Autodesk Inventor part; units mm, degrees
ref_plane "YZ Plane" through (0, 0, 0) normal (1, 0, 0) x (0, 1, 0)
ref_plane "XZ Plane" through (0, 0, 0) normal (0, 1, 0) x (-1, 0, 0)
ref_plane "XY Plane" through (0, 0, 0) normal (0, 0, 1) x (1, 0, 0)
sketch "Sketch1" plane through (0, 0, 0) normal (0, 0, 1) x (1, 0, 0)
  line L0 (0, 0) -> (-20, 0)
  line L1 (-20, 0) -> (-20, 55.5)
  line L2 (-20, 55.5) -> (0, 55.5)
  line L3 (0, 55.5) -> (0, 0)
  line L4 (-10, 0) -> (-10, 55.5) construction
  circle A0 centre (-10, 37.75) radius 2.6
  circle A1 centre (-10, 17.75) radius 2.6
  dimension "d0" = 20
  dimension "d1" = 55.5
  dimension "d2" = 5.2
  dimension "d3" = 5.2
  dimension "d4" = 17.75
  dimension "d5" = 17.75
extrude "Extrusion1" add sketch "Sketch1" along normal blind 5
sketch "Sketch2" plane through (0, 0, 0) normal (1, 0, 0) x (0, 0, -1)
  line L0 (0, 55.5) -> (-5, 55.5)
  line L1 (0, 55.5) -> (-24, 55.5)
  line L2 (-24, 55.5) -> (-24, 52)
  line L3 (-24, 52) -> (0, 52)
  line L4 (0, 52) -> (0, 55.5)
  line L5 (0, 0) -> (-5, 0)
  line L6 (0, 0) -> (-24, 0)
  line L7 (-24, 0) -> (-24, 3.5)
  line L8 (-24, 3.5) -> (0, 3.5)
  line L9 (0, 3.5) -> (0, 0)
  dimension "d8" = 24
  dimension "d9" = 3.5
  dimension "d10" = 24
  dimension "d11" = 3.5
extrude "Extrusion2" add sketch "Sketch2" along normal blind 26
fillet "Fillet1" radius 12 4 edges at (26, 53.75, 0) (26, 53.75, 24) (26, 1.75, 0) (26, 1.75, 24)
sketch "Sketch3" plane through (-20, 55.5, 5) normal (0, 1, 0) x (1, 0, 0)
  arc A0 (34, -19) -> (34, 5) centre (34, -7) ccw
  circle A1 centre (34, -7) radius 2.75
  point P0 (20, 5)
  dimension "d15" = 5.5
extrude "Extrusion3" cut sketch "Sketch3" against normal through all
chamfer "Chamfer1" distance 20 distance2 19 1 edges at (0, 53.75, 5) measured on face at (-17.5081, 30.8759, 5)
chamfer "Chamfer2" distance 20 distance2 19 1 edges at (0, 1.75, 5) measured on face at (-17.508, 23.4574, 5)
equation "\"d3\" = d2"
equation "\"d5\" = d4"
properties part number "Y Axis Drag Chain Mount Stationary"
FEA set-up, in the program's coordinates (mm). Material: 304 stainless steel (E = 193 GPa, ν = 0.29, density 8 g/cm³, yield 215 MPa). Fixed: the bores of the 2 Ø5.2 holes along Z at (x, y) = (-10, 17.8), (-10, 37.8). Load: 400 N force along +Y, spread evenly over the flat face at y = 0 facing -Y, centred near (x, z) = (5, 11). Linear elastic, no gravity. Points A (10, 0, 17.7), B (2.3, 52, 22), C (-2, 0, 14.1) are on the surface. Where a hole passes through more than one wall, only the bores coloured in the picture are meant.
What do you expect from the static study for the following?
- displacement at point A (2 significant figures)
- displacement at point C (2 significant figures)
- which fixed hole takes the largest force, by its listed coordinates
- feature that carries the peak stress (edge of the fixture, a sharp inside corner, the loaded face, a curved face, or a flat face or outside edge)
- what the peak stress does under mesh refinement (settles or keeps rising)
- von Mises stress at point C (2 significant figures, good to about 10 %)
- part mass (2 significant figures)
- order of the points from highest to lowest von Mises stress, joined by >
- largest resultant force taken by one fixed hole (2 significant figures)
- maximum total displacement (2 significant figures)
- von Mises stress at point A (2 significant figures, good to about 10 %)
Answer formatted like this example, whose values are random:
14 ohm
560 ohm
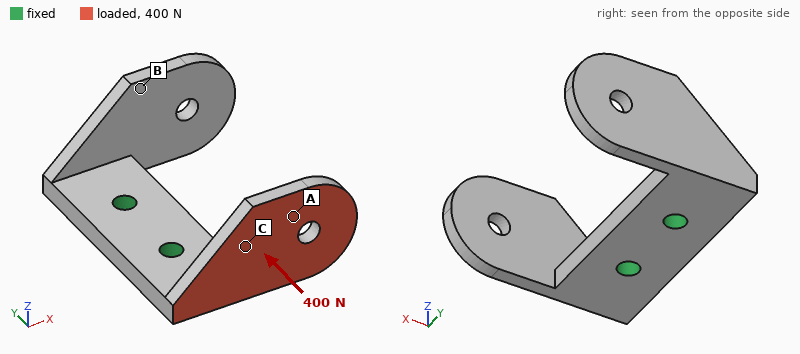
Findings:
0.075 mm
0.034 mm
(-10, 17.8)
a sharp inside corner
keeps rising
53 MPa
83 g
C > A > B
390 N
0.12 mm
19 MPa
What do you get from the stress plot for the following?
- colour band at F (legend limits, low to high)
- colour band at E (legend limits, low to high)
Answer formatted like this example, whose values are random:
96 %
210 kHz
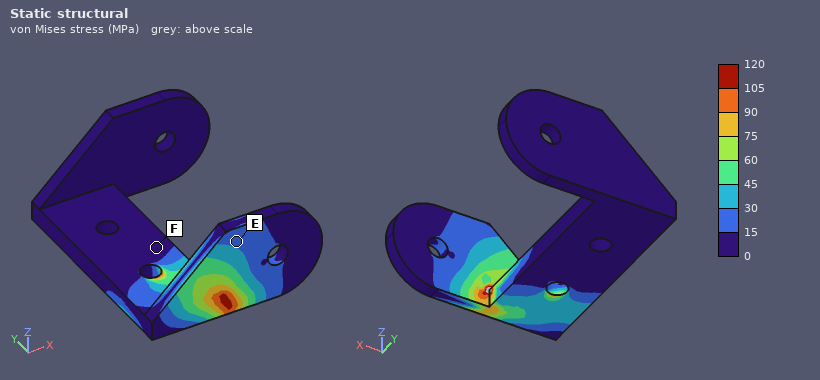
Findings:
0 to 15 MPa
15 to 30 MPa
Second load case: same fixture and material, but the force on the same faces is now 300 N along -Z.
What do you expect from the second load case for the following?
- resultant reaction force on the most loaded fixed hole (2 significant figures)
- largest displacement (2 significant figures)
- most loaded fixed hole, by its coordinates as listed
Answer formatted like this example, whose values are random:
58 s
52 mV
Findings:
350 N
69 µm
(-10, 17.8)
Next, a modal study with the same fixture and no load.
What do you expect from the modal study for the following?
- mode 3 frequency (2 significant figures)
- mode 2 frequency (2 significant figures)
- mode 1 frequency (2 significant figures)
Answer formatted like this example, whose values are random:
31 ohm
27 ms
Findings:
3000 Hz
2300 Hz
2300 Hz
